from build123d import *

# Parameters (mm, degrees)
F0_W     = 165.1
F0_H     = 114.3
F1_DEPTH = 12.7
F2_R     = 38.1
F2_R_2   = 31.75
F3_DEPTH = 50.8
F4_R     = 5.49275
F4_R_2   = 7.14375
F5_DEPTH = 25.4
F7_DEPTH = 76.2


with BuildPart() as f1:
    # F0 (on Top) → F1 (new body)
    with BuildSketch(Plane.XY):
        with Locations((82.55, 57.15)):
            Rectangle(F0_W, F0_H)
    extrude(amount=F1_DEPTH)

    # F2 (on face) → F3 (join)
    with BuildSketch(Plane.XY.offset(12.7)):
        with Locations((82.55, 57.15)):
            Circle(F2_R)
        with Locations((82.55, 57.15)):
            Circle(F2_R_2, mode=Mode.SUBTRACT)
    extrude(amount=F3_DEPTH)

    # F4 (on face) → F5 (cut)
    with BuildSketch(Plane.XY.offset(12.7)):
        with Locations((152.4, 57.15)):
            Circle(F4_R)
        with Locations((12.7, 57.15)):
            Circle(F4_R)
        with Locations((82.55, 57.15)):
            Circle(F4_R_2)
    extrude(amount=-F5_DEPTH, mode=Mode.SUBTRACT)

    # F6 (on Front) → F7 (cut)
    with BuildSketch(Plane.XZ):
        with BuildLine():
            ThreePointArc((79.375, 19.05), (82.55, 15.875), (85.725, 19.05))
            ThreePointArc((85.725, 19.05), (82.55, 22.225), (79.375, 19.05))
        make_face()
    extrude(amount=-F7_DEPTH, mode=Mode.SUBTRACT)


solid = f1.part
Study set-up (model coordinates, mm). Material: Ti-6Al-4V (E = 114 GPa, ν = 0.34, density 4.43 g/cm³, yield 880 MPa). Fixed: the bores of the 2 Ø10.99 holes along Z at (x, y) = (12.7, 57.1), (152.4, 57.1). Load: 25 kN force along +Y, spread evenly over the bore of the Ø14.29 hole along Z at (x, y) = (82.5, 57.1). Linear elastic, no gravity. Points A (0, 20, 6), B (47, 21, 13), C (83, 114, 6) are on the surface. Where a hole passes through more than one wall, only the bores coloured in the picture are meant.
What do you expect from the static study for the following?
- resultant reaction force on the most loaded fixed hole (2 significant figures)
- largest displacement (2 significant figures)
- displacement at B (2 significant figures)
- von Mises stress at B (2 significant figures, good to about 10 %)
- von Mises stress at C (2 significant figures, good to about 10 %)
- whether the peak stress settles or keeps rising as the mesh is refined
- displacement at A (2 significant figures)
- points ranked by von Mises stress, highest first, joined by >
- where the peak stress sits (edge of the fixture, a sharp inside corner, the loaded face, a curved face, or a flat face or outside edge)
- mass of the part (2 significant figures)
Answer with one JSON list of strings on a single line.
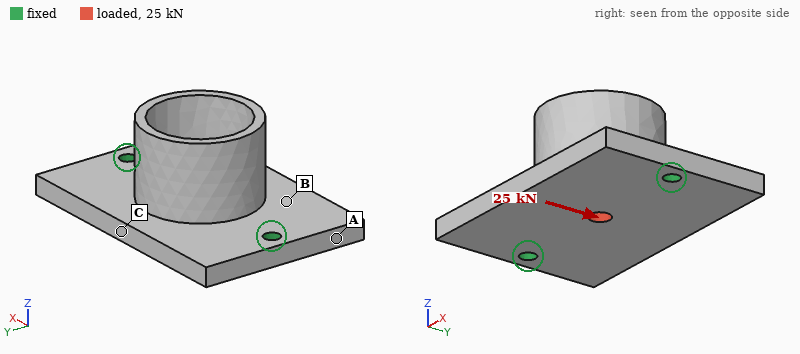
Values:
["13 kN", "28 µm", "15 µm", "17 MPa", "32 MPa", "keeps rising", "5.2 µm", "C > B > A", "edge of the fixture", "1.4 kg"]
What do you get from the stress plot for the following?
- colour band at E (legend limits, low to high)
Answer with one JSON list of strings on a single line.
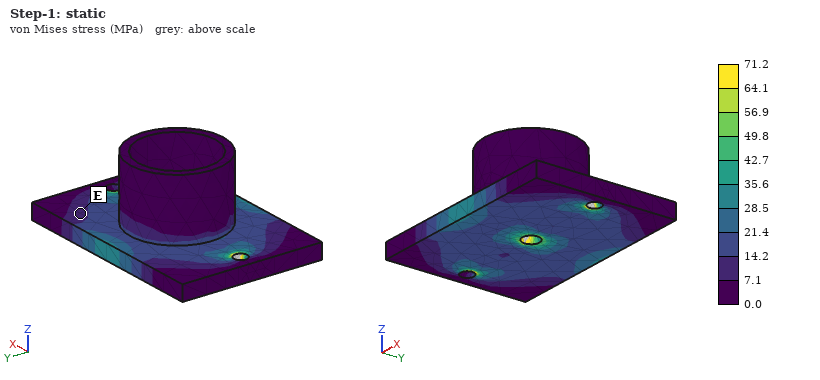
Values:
["7.1 to 14.2 MPa"]
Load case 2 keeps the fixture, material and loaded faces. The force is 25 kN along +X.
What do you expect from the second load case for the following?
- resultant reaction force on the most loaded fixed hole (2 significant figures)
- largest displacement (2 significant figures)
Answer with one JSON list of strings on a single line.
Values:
["13 kN", "16 µm"]
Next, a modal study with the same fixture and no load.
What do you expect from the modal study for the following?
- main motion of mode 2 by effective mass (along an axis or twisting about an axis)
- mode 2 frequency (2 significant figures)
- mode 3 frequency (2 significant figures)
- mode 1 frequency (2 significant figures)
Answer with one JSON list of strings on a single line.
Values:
["along Z", "2300 Hz", "3800 Hz", "1400 Hz"]
